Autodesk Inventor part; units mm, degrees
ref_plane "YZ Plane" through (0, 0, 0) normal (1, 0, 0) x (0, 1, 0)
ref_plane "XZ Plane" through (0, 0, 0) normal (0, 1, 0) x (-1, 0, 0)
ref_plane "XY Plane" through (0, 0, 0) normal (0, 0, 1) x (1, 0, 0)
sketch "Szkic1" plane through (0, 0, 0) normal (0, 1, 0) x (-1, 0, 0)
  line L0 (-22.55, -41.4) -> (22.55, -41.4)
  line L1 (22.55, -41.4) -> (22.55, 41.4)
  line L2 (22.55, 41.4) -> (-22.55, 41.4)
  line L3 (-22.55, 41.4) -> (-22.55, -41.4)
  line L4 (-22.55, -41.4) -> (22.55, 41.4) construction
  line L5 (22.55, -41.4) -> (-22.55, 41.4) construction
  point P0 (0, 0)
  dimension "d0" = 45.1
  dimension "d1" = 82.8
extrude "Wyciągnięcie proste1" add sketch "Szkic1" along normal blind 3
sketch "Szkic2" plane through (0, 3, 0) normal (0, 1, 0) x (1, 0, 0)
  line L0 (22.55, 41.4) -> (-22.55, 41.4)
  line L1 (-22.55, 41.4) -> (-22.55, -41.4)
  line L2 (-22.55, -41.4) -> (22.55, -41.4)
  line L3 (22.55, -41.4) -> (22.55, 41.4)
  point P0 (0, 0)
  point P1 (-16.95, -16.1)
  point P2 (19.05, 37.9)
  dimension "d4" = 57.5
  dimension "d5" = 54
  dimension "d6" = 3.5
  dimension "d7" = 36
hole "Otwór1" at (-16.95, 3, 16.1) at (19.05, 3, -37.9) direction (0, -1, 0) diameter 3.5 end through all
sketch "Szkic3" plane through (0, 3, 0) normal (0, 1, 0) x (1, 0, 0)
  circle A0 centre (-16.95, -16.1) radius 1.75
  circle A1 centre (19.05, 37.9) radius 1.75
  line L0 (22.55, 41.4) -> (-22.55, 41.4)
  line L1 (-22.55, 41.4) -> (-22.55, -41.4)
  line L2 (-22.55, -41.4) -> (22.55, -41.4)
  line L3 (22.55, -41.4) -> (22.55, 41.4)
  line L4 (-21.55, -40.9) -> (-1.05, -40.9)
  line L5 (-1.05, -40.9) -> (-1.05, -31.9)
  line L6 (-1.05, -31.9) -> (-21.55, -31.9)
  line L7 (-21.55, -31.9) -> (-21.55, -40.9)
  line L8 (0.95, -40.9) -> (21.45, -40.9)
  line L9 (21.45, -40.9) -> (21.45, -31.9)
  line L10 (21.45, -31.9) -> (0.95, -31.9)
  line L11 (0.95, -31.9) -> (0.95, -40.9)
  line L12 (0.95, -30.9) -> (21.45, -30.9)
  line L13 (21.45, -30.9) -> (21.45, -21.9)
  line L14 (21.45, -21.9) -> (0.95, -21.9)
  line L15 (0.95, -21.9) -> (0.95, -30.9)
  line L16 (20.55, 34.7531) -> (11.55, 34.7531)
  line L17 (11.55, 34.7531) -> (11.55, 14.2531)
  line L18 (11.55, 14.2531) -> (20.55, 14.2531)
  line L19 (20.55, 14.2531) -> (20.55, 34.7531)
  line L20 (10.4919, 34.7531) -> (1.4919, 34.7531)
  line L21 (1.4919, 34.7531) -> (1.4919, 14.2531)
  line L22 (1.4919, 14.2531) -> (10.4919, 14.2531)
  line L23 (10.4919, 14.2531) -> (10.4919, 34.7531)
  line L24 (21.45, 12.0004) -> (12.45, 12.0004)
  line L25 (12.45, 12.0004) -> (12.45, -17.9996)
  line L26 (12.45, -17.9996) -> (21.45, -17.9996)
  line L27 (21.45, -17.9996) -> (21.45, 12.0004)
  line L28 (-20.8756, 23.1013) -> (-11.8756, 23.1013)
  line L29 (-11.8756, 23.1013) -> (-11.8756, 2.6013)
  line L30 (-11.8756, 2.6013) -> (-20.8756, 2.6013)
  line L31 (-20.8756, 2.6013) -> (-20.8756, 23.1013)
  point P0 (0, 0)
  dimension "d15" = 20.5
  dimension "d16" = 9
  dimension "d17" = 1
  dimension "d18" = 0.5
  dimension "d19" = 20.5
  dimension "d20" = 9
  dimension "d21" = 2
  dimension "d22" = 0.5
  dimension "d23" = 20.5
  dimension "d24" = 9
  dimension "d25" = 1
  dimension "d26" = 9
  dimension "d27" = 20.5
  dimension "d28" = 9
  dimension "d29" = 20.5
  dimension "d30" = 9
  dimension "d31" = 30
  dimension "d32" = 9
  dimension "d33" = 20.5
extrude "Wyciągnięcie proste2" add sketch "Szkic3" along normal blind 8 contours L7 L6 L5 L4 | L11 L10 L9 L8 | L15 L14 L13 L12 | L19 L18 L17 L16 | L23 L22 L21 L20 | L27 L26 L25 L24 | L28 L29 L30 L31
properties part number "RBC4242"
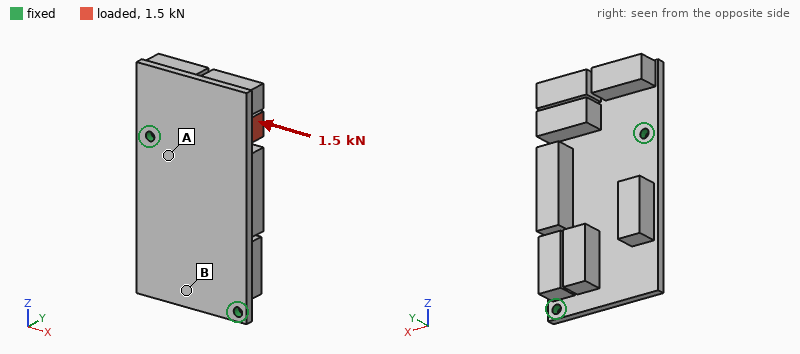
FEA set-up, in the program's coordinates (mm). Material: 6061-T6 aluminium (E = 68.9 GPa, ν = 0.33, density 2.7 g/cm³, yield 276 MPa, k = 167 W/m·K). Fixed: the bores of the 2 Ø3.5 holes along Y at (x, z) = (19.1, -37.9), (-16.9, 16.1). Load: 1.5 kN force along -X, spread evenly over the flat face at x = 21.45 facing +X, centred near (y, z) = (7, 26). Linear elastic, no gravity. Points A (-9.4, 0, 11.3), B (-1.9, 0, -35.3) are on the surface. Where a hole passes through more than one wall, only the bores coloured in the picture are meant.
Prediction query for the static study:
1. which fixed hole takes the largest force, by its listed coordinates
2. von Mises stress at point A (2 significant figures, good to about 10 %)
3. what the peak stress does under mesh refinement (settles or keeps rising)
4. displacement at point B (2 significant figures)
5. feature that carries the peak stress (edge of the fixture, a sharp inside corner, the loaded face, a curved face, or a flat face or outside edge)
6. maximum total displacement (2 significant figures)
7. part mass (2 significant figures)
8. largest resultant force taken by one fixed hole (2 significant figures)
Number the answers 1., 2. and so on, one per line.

1. (-16.9, 16.1)
2. 37 MPa
3. keeps rising
4. 0.082 mm
5. edge of the fixture
6. 0.46 mm
7. 60 g
8. 1.5 kN
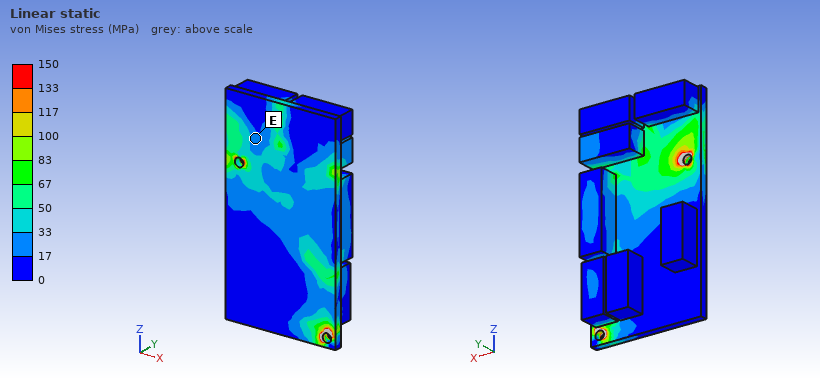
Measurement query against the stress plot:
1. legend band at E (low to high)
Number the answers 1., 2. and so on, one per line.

1. 17 to 33 MPa
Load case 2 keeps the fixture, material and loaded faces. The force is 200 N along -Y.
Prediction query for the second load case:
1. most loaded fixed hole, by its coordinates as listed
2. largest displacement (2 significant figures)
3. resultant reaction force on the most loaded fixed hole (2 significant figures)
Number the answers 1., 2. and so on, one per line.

1. (-16.9, 16.1)
2. 0.44 mm
3. 170 N
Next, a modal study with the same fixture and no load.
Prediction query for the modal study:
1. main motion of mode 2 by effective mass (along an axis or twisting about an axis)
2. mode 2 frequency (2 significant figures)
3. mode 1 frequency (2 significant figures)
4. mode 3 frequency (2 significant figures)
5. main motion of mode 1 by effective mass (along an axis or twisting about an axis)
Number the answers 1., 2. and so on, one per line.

1. along Y
2. 2100 Hz
3. 1000 Hz
4. 2500 Hz
5. along Y
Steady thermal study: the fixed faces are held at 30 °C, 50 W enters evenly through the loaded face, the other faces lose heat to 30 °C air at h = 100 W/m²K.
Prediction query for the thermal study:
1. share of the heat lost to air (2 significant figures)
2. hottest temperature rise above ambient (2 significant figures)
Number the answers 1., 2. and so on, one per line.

1. 46 %
2. 77 K
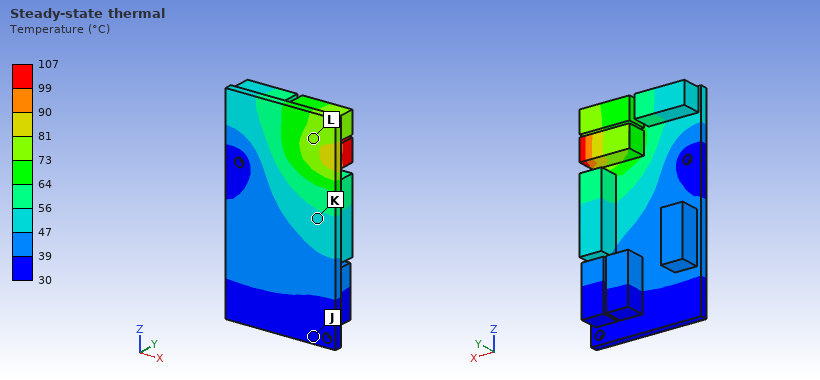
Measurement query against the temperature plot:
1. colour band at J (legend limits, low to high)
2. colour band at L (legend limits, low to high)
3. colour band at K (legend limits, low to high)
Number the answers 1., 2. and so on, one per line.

1. 30 to 39 °C
2. 73 to 81 °C
3. 47 to 56 °C
